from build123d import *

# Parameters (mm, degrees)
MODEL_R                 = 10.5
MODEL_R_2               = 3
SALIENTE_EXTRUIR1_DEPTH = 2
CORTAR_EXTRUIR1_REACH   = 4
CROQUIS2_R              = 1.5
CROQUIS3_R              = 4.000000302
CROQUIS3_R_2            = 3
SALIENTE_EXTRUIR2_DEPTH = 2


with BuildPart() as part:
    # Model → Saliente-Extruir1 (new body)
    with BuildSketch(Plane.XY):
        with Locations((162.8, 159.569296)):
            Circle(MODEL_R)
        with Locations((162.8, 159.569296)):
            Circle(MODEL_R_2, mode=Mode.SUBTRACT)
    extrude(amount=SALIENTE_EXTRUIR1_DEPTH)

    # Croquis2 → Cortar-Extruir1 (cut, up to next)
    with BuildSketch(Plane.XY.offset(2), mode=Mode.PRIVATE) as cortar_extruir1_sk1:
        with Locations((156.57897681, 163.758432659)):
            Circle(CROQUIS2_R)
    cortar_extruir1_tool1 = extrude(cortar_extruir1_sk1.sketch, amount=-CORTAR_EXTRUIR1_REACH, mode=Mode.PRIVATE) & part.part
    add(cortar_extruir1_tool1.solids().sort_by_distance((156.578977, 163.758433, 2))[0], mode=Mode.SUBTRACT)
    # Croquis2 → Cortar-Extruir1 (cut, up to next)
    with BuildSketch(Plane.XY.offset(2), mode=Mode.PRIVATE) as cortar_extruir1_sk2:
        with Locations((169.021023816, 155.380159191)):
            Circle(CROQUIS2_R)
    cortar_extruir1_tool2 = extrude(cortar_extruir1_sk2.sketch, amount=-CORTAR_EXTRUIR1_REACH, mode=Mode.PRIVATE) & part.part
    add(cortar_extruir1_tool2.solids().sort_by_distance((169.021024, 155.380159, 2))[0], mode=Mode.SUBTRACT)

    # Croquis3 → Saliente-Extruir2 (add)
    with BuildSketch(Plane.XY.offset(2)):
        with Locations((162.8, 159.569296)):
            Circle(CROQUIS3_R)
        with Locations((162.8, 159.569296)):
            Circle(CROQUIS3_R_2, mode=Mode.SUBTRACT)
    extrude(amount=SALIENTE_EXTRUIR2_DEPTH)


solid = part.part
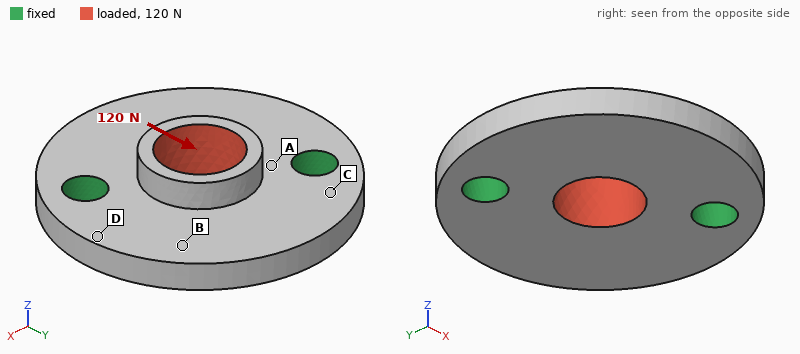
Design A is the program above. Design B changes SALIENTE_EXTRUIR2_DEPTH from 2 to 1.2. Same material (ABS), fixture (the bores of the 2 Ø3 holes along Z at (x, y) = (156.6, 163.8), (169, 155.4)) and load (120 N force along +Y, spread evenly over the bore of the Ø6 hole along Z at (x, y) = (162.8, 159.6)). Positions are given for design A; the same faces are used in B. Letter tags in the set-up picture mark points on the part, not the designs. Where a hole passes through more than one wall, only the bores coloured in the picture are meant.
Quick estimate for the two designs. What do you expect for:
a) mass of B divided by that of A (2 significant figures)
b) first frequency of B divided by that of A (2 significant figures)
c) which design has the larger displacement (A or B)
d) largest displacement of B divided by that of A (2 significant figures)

0.97
1.00
A
0.64
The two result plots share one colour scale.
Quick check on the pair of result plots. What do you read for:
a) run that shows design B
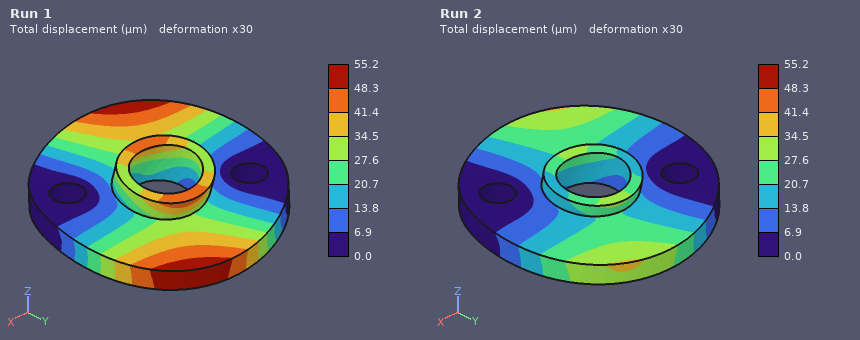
Run 2
